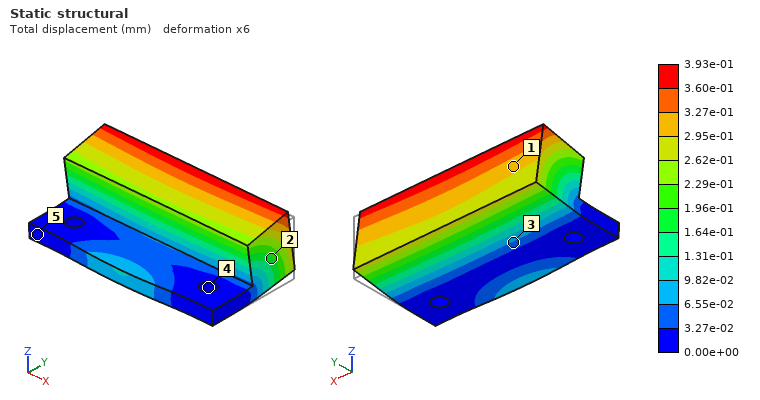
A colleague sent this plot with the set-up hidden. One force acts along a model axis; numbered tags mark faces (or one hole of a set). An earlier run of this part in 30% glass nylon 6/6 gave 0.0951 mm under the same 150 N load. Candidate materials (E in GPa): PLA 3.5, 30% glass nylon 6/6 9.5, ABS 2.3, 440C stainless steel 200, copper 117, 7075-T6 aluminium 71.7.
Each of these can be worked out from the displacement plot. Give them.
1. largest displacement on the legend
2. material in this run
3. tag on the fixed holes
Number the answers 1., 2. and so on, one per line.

1. 3.93e-01 mm
2. ABS
3. 4
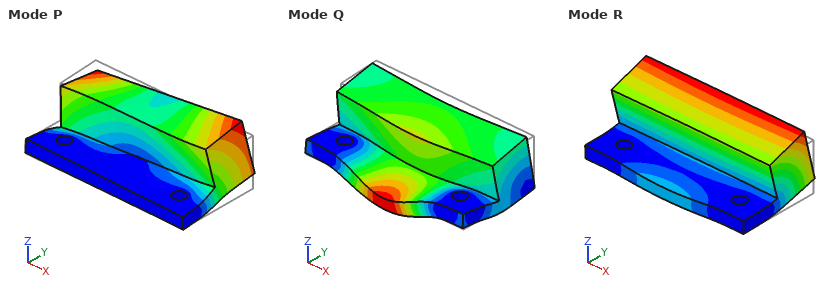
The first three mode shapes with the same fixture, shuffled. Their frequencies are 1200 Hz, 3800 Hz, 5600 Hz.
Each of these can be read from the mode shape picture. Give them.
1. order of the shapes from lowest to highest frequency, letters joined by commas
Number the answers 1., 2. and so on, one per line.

1. R, P, Q
